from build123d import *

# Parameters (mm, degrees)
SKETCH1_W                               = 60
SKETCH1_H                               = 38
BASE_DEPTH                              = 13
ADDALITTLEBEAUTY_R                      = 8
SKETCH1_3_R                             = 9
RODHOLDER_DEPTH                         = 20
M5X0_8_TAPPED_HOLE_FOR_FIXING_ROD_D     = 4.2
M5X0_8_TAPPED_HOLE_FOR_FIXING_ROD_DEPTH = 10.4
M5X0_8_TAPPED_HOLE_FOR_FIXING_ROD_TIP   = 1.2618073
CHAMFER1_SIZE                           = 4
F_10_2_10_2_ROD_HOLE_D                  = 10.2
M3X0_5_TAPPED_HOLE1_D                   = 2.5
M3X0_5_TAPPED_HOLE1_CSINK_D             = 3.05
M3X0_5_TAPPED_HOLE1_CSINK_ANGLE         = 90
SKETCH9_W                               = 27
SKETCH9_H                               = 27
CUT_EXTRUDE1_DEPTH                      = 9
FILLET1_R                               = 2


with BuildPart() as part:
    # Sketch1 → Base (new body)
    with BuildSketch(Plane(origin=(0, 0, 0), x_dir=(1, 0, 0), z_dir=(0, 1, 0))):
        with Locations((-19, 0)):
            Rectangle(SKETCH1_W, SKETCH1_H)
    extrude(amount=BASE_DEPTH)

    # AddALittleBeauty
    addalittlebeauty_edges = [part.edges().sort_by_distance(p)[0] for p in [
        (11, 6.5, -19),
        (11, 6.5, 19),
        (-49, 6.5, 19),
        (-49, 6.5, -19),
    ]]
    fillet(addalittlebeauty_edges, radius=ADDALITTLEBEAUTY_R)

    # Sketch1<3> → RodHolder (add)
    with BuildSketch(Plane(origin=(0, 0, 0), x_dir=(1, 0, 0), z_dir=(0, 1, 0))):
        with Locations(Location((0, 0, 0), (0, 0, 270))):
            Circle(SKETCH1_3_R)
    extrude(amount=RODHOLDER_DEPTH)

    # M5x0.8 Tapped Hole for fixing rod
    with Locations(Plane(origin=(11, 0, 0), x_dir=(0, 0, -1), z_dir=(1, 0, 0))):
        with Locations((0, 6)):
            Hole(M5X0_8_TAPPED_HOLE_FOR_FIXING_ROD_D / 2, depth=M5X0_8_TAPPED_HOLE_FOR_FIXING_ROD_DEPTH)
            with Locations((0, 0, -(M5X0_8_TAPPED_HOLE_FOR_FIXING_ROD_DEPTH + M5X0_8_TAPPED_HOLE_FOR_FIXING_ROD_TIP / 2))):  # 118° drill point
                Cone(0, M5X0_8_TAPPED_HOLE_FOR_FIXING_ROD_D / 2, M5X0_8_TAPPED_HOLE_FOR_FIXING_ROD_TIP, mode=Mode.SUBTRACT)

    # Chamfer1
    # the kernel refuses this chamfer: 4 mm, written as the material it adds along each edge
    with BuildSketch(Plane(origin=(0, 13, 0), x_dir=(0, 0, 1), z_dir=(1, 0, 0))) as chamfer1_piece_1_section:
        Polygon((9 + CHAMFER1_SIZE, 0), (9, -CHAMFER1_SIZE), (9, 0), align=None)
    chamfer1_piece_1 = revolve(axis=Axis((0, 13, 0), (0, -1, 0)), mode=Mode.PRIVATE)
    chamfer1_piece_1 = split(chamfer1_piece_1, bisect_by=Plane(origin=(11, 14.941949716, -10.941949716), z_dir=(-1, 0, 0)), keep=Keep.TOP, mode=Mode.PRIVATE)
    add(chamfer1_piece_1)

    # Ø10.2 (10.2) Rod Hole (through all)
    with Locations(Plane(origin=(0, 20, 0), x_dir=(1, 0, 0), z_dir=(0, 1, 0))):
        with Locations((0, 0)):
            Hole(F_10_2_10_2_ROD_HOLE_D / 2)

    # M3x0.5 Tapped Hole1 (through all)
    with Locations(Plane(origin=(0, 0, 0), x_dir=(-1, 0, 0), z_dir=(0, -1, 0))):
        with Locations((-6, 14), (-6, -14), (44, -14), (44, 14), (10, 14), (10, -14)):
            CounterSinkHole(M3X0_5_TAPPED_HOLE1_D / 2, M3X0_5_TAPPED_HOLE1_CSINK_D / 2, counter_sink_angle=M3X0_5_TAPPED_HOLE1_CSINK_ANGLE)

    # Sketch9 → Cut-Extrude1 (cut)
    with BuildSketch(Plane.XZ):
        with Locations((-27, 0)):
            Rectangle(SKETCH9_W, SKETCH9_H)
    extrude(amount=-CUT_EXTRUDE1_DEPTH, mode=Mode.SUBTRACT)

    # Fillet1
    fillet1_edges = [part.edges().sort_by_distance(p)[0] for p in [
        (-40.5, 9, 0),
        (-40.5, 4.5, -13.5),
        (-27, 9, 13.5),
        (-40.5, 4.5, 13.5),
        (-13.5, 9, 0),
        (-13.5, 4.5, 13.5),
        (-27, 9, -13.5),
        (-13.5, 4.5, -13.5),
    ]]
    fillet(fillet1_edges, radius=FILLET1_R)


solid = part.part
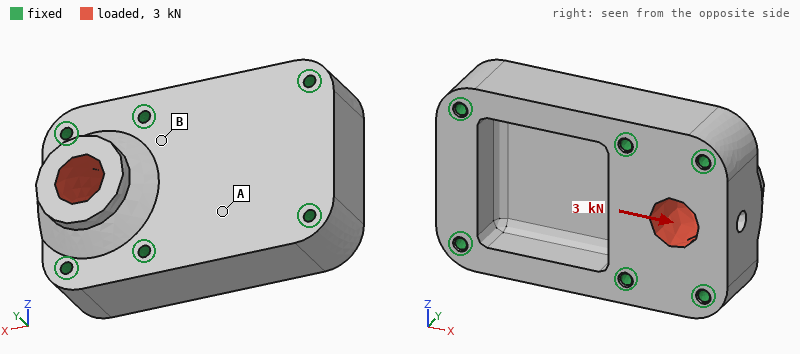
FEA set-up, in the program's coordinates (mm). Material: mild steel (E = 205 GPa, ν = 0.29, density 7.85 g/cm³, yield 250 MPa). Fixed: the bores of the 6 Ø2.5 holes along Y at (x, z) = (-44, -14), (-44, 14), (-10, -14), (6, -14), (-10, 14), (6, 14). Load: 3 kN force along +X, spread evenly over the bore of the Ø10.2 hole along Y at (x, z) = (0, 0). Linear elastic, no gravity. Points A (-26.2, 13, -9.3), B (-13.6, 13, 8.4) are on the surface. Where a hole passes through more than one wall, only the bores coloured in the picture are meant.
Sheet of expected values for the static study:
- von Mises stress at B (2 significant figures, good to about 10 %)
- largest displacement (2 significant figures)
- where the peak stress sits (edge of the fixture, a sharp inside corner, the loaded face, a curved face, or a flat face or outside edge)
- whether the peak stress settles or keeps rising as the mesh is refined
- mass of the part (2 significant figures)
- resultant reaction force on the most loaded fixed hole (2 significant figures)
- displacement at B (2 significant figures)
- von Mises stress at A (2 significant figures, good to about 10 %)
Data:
6.8 MPa
1.6 µm
edge of the fixture
keeps rising
180 g
850 N
0.33 µm
2.5 MPa
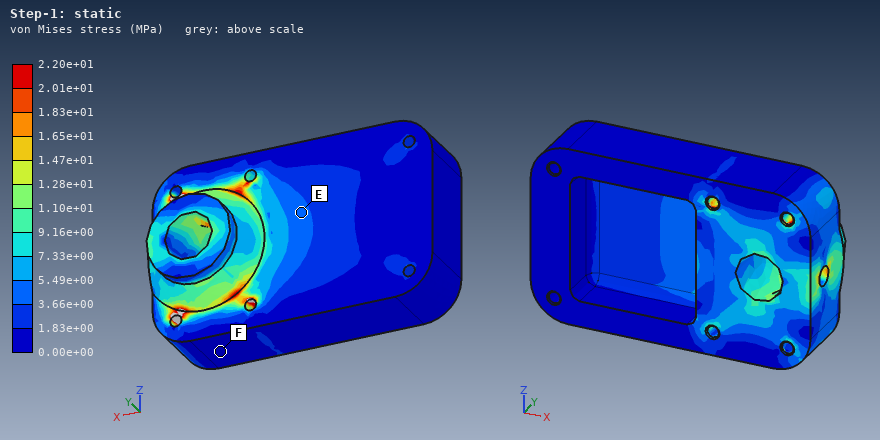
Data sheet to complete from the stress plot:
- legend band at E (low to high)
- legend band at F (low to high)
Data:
3.66e+00 to 5.49e+00 MPa
0.00e+00 to 1.83e+00 MPa
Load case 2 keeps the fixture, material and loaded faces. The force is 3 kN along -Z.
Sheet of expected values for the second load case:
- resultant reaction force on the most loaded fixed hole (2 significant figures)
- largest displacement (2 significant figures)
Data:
870 N
0.88 µm
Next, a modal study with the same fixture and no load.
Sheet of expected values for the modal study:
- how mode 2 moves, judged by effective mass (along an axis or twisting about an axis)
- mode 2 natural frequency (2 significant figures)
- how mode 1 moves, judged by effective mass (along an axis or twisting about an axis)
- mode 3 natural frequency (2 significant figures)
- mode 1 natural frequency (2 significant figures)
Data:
along Z
33 kHz
along Y
34 kHz
26 kHz
